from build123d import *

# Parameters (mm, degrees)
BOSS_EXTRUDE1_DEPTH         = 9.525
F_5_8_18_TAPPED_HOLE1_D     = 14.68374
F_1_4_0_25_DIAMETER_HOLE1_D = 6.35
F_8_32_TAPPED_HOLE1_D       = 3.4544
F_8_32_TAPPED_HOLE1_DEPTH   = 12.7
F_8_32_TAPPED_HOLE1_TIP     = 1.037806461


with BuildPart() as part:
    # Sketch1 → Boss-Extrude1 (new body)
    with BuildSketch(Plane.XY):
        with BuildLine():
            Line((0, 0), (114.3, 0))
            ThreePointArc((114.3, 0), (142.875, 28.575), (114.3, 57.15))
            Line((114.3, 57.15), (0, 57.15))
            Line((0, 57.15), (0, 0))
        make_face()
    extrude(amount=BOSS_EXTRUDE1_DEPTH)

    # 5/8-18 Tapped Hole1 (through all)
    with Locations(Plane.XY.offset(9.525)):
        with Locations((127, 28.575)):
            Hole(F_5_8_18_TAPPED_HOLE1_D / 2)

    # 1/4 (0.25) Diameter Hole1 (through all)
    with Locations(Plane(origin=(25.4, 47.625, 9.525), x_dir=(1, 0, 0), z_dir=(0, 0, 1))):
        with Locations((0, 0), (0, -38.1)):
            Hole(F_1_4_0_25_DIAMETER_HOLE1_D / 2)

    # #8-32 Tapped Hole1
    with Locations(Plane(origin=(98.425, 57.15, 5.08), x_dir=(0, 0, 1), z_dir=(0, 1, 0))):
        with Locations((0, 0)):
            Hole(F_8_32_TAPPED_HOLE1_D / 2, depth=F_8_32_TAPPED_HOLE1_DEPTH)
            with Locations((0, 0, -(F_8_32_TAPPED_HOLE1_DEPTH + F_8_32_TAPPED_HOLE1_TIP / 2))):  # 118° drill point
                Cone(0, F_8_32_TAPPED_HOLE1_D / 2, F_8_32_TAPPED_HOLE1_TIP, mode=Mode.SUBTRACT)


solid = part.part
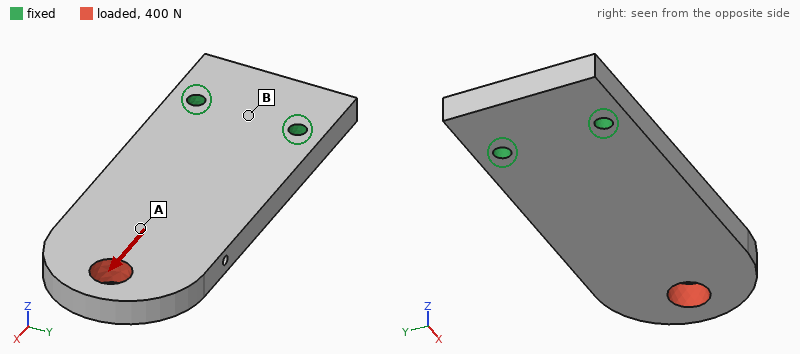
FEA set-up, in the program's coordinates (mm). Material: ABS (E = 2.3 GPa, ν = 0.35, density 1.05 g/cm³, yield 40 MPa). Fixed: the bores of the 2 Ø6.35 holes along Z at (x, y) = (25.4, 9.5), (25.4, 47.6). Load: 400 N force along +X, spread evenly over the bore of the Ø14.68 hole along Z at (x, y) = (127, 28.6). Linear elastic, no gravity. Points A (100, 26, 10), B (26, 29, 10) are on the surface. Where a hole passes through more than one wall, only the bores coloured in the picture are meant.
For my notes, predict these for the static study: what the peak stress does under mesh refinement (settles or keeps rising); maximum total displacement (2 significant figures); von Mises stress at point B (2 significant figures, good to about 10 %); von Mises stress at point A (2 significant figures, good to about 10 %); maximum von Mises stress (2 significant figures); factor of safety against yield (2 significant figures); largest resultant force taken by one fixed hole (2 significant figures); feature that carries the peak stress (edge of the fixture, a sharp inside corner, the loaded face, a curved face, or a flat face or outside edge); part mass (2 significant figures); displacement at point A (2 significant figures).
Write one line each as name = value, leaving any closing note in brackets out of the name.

what the peak stress does under mesh refinement = settles
maximum total displacement = 50 µm
von Mises stress at point B = 0.27 MPa
von Mises stress at point A = 0.90 MPa
maximum von Mises stress = 2.7 MPa
factor of safety against yield = 15
largest resultant force taken by one fixed hole = 200 N
feature that carries the peak stress = the loaded face
part mass = 76 g
displacement at point A = 26 µm
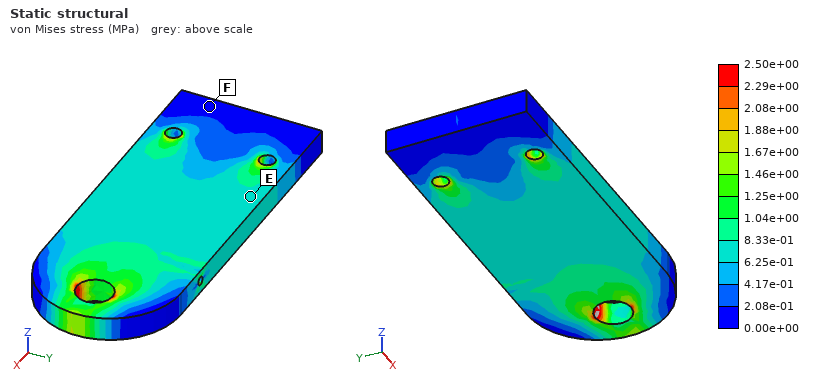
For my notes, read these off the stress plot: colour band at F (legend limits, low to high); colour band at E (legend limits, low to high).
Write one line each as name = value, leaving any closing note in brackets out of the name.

colour band at F = 0.00e+00 to 2.08e-01 MPa
colour band at E = 6.25e-01 to 8.33e-01 MPa
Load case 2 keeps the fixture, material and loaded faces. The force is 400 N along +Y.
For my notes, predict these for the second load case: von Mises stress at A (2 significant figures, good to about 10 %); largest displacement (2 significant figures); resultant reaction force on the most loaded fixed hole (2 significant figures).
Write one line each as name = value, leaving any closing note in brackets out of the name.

von Mises stress at A = 2.1 MPa
largest displacement = 0.64 mm
resultant reaction force on the most loaded fixed hole = 1.0 kN
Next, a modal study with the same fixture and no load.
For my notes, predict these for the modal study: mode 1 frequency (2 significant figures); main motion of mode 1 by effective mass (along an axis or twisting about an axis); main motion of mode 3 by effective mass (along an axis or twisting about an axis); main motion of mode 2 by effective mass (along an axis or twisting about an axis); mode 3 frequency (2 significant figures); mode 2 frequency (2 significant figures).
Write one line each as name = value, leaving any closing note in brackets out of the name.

mode 1 frequency = 190 Hz
main motion of mode 1 by effective mass = along Z
main motion of mode 3 by effective mass = along Y
main motion of mode 2 by effective mass = twisting about X
mode 3 frequency = 940 Hz
mode 2 frequency = 770 Hz
